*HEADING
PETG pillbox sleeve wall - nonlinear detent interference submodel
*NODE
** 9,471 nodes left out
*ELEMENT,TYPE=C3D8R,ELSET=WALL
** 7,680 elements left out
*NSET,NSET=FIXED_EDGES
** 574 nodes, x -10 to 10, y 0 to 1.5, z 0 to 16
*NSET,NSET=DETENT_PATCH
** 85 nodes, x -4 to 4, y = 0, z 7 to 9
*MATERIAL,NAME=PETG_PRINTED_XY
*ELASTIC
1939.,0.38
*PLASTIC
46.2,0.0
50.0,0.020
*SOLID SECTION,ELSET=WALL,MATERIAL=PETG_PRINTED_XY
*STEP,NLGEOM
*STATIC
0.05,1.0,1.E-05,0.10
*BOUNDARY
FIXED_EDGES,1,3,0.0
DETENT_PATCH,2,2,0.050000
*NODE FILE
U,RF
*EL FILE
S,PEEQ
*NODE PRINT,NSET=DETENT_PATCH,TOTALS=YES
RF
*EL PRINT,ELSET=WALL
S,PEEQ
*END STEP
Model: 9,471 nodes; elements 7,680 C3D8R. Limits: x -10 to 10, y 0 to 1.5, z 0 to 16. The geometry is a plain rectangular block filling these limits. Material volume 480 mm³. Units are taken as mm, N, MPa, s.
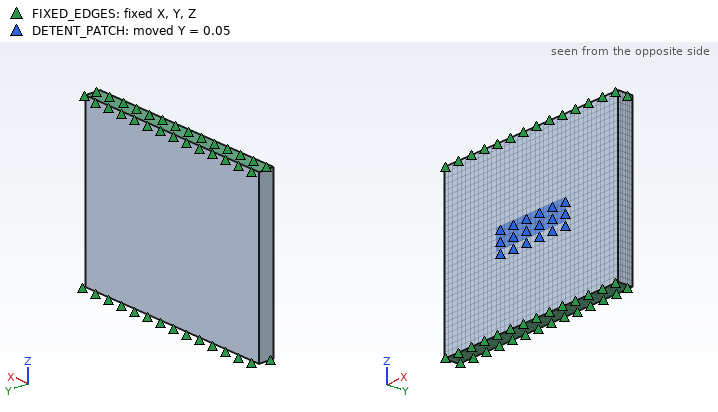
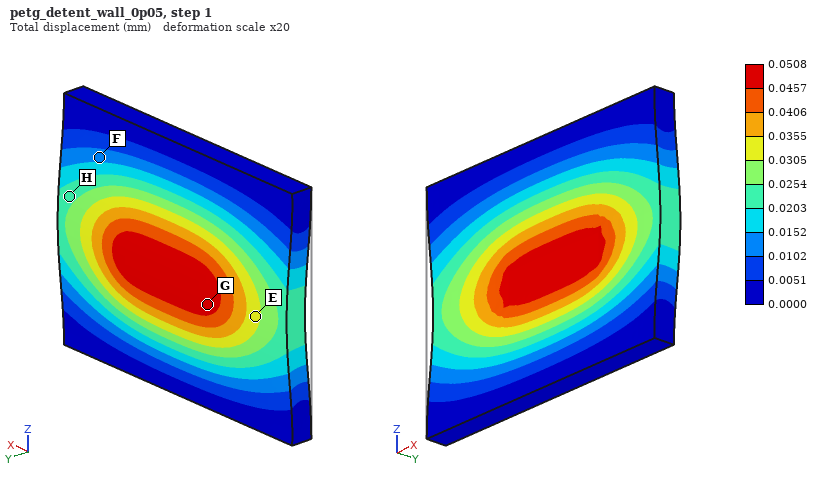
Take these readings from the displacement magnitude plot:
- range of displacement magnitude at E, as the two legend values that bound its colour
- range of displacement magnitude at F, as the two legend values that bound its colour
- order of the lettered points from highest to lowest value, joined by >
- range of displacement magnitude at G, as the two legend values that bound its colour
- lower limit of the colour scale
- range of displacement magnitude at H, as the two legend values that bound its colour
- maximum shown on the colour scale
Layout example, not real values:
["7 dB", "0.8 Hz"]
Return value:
["0.0305 to 0.0355 mm", "0.0102 to 0.0152 mm", "G > E > H > F", "0.0457 to 0.0508 mm", "0.0000 mm", "0.0203 to 0.0254 mm", "0.0508 mm"]
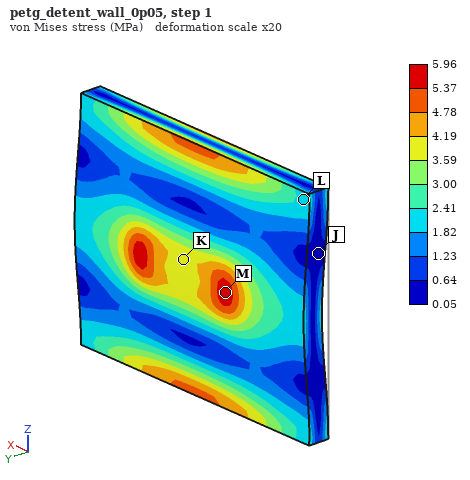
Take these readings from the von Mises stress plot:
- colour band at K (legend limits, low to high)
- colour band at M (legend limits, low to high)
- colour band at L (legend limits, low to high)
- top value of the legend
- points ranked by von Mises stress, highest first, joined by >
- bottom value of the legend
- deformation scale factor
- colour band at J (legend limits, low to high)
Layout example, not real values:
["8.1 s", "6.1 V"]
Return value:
["3.59 to 4.19 MPa", "5.37 to 5.96 MPa", "1.82 to 2.41 MPa", "5.96 MPa", "M > K > L > J", "0.05 MPa", "20", "0.05 to 0.64 MPa"]
